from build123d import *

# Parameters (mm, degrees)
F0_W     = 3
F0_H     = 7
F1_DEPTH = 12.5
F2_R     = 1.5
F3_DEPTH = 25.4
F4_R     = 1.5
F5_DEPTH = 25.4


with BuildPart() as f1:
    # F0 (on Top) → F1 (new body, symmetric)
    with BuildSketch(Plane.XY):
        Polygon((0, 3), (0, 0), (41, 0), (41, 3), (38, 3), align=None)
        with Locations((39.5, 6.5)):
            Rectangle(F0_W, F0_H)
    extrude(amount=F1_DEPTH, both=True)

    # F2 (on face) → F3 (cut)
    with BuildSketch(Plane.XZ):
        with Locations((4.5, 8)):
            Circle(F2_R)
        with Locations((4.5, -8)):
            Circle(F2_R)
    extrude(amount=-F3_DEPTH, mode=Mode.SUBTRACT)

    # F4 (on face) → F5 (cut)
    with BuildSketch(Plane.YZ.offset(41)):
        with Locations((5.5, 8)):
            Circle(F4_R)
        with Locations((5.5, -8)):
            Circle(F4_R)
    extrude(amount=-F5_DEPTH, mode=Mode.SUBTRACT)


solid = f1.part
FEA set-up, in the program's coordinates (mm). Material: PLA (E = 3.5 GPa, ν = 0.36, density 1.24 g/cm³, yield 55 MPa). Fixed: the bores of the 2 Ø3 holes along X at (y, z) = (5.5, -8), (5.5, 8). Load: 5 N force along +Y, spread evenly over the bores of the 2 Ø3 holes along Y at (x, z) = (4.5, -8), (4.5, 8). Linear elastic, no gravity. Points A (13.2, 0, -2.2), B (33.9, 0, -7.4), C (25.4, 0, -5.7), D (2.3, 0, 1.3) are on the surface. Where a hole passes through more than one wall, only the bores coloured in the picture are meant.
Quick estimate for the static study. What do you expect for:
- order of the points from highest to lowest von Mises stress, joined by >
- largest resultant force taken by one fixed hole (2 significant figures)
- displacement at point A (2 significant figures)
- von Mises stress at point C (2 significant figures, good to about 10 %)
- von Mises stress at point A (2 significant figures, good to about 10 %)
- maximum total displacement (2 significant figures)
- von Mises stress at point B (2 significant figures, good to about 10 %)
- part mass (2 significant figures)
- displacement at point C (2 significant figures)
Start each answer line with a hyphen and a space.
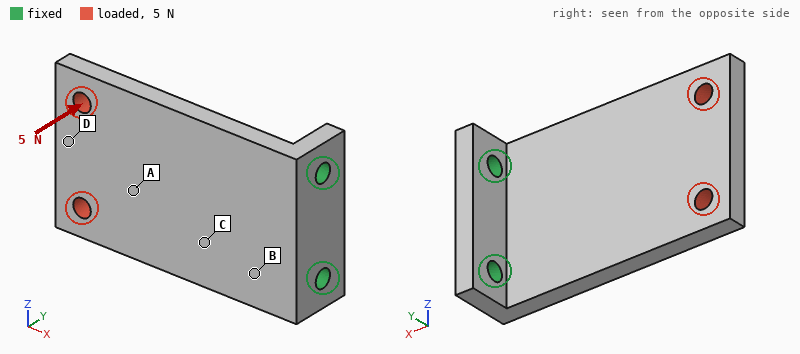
- B > C > A > D
- 3.0 N
- 0.29 mm
- 2.6 MPa
- 1.1 MPa
- 0.51 mm
- 3.7 MPa
- 4.4 g
- 0.11 mm
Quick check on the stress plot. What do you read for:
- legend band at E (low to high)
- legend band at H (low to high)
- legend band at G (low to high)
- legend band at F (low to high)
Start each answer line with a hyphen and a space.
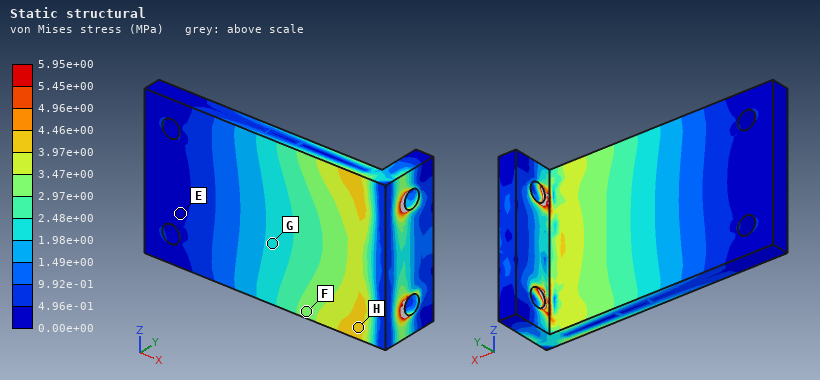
- 0.00e+00 to 4.96e-01 MPa
- 3.97e+00 to 4.46e+00 MPa
- 1.98e+00 to 2.48e+00 MPa
- 2.97e+00 to 3.47e+00 MPa
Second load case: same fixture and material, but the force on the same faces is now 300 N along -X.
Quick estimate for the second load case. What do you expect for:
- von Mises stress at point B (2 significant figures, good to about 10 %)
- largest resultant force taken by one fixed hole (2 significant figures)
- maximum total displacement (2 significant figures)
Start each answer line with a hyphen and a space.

- 4.9 MPa
- 150 N
- 0.50 mm
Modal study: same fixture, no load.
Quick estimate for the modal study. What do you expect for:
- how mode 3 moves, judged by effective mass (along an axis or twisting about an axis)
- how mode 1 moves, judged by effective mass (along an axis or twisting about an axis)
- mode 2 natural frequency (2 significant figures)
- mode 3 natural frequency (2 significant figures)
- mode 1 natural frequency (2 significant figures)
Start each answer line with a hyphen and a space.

- along Z
- along Y
- 1700 Hz
- 2400 Hz
- 480 Hz
